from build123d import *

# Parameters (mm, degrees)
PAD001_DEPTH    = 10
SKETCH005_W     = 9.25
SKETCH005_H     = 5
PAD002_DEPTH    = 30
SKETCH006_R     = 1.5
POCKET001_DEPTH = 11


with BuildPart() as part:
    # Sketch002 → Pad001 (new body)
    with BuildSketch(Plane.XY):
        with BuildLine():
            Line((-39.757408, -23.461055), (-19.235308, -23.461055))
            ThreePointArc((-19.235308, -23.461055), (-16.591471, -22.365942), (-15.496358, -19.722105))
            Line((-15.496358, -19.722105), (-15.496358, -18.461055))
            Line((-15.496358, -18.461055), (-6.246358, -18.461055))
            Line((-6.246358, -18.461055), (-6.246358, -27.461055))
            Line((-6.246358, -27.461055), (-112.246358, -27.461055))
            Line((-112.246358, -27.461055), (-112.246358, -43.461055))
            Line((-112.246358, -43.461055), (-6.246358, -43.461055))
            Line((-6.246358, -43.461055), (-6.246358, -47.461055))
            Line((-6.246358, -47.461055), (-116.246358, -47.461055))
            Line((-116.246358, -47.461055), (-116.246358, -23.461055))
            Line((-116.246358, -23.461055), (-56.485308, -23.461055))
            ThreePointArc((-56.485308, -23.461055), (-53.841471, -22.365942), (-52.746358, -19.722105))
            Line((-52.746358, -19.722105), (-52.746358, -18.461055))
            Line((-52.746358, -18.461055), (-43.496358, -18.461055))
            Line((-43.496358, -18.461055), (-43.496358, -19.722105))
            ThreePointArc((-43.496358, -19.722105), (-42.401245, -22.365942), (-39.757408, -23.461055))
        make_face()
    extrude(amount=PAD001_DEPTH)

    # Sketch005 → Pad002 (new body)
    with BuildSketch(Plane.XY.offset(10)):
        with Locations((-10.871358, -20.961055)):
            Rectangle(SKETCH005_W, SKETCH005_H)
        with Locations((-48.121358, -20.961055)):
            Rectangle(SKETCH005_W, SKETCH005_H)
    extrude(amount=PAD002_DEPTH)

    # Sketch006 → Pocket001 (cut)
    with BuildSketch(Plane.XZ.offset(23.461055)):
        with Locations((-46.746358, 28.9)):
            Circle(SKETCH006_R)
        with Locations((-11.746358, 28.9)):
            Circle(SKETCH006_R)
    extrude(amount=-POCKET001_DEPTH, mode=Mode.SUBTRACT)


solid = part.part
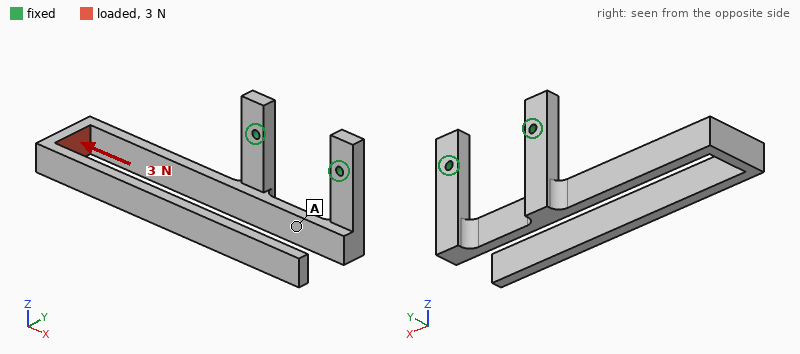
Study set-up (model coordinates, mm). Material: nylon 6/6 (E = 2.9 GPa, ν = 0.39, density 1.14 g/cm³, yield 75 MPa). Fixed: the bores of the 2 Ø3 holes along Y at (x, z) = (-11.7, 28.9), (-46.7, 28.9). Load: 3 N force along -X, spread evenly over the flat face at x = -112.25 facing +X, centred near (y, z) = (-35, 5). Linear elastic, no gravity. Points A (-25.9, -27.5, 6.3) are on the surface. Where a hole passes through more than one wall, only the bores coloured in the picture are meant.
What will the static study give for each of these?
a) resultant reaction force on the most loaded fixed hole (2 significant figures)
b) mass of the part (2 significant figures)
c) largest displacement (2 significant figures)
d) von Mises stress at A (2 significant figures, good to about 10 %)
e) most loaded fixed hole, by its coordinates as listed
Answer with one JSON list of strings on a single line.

["2.4 N", "15 g", "1.1 mm", "0.27 MPa", "(-11.7, 28.9)"]
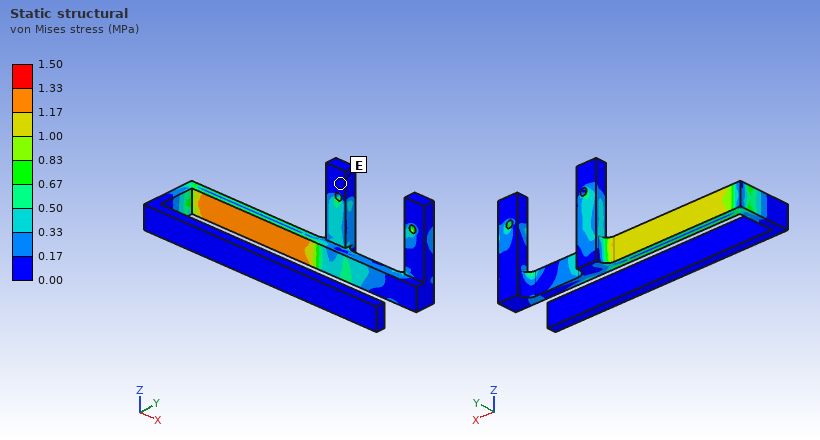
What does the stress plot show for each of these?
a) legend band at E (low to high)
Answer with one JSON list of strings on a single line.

["0.00 to 0.17 MPa"]
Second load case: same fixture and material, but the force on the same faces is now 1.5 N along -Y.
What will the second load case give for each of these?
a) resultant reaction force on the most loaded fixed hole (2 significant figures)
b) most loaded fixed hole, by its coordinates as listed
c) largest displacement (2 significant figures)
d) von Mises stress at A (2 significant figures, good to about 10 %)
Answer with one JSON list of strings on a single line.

["3.4 N", "(-46.7, 28.9)", "1.3 mm", "0.83 MPa"]
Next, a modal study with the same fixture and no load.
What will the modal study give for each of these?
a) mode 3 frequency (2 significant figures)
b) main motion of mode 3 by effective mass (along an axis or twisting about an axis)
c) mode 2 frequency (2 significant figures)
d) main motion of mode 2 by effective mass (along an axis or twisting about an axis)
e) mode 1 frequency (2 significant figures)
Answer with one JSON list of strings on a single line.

["110 Hz", "along Y", "84 Hz", "along Z", "53 Hz"]
